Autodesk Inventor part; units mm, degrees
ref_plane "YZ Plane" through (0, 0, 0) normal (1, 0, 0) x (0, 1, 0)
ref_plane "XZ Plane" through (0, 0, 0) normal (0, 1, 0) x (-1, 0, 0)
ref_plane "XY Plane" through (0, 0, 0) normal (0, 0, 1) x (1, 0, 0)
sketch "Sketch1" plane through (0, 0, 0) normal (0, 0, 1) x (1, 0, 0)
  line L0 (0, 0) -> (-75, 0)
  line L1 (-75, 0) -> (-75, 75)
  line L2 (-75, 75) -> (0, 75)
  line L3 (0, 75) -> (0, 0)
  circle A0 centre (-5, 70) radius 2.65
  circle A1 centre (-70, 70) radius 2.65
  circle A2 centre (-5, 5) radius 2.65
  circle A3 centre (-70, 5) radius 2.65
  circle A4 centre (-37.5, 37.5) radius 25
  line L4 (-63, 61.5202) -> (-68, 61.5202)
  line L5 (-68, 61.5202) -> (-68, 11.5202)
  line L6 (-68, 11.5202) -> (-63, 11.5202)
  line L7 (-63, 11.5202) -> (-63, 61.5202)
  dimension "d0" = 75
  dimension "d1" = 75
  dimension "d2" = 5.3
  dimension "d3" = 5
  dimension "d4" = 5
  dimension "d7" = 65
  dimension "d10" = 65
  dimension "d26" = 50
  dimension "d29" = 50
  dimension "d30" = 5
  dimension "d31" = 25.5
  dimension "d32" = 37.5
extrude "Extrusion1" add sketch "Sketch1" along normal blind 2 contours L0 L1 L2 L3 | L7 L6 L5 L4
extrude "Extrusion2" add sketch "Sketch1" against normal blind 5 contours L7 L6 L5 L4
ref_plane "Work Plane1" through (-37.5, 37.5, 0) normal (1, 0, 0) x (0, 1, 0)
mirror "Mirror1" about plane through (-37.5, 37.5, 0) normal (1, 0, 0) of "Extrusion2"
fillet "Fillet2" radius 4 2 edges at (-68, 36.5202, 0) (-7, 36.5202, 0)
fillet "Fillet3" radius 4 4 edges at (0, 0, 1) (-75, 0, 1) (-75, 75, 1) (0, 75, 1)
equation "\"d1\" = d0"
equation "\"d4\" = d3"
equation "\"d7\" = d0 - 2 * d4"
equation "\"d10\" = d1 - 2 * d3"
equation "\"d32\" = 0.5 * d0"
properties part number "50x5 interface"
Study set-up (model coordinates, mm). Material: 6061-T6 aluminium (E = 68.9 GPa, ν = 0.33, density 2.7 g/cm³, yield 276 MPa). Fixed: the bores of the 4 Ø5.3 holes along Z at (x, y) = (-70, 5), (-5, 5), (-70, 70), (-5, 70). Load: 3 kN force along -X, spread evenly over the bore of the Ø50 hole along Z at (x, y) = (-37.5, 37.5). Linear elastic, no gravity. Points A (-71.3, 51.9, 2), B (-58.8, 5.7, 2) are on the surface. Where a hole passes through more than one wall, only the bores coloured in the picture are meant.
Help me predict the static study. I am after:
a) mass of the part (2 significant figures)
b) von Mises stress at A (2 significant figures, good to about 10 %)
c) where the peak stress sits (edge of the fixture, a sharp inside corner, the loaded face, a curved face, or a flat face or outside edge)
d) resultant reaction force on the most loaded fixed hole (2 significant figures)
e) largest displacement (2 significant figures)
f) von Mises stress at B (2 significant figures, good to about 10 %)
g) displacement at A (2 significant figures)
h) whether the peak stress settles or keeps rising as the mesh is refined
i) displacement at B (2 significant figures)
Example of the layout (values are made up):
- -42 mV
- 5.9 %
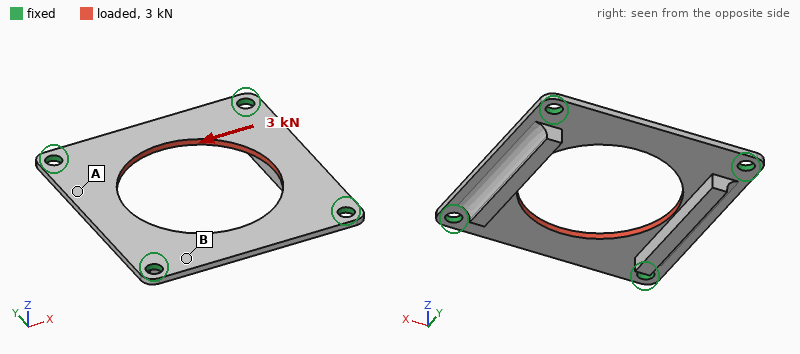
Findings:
- 27 g
- 15 MPa
- edge of the fixture
- 790 N
- 29 µm
- 23 MPa
- 18 µm
- keeps rising
- 5.8 µm
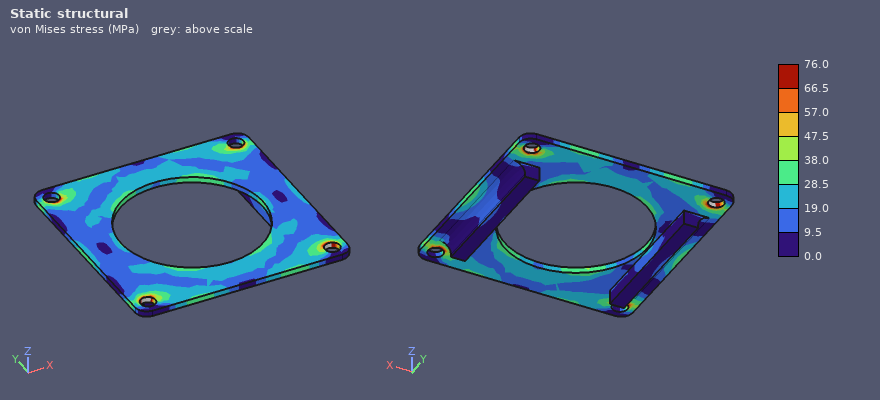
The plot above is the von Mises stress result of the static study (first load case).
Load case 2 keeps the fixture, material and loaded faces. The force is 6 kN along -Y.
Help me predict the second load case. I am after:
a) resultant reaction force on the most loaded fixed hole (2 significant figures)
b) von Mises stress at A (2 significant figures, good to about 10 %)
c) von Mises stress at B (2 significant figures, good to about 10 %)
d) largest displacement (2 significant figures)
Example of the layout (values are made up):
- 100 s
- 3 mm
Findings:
- 1.6 kN
- 40 MPa
- 28 MPa
- 56 µm
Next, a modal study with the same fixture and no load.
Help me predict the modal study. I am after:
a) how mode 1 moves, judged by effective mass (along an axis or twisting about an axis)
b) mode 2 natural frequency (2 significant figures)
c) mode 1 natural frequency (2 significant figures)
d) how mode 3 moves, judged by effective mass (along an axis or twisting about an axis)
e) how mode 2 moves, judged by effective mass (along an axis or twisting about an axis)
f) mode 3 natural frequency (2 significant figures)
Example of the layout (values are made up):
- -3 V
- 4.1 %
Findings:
- along Z
- 3300 Hz
- 2900 Hz
- along Z
- twisting about X
- 4800 Hz
